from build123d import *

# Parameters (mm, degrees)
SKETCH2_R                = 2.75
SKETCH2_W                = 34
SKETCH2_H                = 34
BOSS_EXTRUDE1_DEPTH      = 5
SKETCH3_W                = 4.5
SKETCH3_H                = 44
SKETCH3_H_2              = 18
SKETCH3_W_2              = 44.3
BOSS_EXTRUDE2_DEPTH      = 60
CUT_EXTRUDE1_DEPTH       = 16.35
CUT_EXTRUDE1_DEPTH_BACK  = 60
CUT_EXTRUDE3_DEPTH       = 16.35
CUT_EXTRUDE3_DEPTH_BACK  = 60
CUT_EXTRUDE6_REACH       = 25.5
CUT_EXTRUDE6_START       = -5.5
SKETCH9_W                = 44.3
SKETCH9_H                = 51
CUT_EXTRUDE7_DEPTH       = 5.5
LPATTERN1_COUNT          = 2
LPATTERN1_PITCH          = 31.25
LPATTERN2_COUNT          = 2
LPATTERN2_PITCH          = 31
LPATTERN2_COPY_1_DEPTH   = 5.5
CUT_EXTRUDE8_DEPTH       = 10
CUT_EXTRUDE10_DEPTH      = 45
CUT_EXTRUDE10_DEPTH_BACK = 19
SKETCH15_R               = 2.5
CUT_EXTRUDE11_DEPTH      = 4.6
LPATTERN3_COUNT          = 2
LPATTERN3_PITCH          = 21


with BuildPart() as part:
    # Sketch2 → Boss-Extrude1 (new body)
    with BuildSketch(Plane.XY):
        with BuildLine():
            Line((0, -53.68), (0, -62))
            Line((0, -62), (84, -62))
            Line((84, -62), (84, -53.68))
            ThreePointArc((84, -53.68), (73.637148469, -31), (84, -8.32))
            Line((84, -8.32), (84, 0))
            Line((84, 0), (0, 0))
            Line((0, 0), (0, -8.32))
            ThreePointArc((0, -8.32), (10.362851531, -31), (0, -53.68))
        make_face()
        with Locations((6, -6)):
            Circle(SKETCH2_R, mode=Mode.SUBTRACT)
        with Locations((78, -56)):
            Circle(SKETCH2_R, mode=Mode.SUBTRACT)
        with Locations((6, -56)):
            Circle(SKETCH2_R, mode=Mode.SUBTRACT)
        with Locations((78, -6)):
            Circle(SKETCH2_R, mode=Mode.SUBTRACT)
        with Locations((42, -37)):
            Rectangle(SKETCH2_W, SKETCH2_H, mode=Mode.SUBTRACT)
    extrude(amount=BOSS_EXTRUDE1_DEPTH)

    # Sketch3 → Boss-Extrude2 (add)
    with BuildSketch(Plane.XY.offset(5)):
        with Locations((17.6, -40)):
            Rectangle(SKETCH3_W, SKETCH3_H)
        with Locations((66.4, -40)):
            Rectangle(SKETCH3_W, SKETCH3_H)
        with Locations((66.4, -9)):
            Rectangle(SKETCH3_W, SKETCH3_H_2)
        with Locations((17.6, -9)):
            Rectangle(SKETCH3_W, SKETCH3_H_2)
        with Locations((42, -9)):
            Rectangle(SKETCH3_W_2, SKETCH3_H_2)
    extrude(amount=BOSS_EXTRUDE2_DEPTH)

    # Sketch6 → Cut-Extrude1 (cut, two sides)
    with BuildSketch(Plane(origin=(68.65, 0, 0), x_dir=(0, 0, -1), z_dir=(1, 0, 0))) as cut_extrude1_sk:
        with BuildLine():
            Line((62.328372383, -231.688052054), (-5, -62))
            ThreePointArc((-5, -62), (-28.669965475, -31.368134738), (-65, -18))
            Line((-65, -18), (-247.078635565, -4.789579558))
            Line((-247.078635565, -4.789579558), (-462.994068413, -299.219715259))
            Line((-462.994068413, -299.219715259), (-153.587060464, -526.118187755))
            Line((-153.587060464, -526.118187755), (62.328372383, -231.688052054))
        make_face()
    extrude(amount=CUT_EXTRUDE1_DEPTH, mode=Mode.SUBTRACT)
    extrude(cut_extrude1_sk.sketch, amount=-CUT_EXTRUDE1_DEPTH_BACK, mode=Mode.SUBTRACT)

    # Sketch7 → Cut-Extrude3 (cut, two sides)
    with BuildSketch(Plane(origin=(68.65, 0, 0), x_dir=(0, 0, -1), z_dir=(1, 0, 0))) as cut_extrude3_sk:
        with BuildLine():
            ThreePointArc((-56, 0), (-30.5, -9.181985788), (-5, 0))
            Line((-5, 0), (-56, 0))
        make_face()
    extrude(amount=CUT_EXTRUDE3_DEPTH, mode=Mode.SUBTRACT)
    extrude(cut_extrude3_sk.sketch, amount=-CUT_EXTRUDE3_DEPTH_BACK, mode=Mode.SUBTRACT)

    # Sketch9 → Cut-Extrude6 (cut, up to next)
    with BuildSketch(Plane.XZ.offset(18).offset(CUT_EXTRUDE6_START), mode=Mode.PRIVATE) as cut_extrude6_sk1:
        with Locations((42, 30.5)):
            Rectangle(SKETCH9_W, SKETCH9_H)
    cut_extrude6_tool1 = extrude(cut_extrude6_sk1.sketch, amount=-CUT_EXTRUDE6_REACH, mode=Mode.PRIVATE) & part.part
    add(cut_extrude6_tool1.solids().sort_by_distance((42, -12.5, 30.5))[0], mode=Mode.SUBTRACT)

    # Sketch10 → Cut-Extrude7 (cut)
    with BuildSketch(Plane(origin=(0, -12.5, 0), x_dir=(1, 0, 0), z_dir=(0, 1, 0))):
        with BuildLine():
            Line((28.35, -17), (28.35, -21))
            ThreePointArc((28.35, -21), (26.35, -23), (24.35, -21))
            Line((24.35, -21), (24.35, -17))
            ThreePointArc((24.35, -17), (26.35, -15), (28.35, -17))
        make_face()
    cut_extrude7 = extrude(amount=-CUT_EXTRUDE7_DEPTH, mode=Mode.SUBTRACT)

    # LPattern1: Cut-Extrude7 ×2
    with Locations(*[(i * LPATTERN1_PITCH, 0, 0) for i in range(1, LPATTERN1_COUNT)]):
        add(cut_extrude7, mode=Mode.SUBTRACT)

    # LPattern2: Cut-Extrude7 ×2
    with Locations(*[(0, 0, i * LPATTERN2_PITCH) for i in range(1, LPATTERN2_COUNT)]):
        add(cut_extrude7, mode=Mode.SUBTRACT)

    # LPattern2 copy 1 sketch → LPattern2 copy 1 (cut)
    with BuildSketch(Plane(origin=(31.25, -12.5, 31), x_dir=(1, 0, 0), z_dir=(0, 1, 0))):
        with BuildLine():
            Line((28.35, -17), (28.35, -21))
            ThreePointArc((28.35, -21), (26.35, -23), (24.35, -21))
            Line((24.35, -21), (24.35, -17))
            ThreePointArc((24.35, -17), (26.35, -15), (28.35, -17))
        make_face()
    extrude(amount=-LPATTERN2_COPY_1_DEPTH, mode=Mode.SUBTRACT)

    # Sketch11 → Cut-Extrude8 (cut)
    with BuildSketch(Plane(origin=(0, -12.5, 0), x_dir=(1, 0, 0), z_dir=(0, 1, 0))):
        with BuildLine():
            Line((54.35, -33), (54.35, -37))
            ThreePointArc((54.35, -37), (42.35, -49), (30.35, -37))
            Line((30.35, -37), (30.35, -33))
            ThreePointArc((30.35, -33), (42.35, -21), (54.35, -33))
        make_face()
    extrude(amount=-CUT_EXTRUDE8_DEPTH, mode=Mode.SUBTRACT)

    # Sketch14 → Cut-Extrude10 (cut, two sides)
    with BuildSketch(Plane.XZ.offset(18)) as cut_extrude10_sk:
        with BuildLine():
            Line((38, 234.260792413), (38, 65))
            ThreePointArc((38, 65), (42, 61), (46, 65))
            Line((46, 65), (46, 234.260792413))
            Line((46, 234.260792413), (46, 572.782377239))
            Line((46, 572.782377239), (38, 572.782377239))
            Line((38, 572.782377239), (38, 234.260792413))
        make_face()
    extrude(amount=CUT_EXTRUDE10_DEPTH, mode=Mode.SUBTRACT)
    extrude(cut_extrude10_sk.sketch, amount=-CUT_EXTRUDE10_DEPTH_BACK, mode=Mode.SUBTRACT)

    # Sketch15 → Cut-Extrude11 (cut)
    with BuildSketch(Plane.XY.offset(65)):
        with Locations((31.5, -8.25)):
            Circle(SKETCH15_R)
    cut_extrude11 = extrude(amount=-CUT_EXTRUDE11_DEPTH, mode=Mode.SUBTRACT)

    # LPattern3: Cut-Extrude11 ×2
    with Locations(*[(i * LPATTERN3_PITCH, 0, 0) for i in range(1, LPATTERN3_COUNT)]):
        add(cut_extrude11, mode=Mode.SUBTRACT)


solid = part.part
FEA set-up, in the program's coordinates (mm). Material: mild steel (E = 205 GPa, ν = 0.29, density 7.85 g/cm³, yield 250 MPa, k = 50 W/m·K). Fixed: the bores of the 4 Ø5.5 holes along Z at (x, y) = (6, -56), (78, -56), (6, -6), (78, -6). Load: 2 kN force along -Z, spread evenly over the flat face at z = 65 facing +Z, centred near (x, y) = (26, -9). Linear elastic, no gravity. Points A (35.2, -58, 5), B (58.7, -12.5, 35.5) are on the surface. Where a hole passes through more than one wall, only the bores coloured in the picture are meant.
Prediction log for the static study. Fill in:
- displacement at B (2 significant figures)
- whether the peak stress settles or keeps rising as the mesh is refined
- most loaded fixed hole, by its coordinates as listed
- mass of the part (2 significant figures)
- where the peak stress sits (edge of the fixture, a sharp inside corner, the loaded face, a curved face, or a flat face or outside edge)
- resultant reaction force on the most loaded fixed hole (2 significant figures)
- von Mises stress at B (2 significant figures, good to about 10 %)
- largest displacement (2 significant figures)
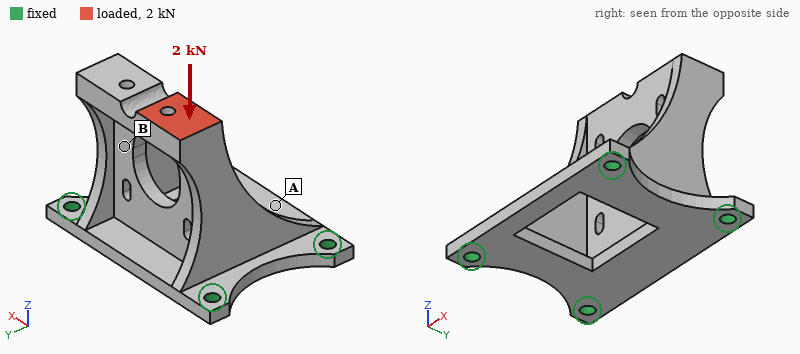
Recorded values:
7.1 µm
keeps rising
(6, -6)
360 g
edge of the fixture
1.4 kN
15 MPa
41 µm
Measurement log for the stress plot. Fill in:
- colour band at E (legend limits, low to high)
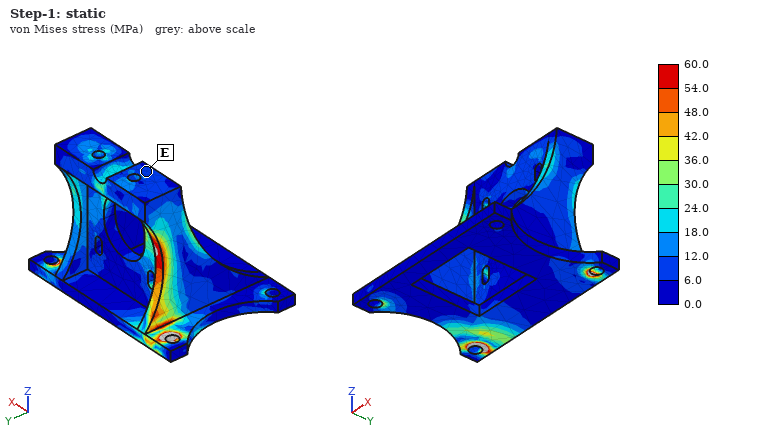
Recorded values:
6.0 to 12.0 MPa
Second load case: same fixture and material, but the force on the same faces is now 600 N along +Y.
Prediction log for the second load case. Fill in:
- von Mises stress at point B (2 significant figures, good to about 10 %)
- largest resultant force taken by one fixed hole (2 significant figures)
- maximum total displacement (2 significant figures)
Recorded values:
12 MPa
610 N
46 µm
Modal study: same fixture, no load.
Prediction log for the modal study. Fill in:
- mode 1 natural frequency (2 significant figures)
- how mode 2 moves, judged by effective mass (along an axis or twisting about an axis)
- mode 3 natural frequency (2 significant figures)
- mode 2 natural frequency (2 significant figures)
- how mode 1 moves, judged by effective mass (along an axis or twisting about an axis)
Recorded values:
2600 Hz
along X
4600 Hz
3800 Hz
along Y
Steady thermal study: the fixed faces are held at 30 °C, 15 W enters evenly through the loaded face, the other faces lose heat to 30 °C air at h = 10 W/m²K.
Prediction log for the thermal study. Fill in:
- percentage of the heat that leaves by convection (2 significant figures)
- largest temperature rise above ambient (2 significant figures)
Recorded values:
28 %
68 K
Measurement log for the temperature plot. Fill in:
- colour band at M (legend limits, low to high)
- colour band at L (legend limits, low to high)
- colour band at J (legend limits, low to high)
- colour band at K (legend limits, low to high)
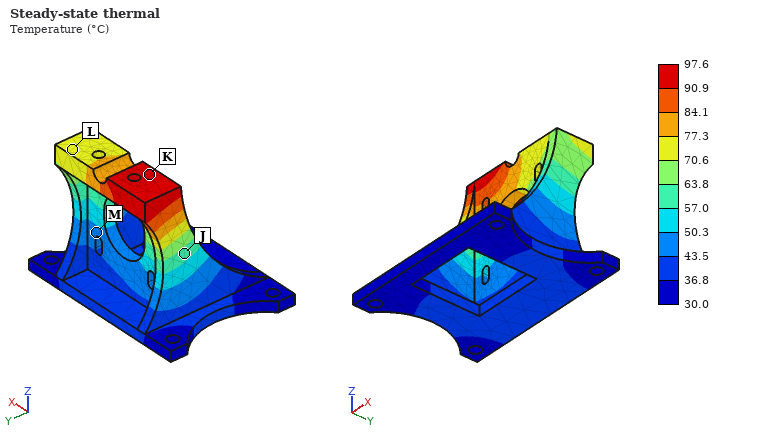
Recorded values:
43.5 to 50.3 °C
70.6 to 77.3 °C
57.0 to 63.8 °C
90.9 to 97.6 °C
